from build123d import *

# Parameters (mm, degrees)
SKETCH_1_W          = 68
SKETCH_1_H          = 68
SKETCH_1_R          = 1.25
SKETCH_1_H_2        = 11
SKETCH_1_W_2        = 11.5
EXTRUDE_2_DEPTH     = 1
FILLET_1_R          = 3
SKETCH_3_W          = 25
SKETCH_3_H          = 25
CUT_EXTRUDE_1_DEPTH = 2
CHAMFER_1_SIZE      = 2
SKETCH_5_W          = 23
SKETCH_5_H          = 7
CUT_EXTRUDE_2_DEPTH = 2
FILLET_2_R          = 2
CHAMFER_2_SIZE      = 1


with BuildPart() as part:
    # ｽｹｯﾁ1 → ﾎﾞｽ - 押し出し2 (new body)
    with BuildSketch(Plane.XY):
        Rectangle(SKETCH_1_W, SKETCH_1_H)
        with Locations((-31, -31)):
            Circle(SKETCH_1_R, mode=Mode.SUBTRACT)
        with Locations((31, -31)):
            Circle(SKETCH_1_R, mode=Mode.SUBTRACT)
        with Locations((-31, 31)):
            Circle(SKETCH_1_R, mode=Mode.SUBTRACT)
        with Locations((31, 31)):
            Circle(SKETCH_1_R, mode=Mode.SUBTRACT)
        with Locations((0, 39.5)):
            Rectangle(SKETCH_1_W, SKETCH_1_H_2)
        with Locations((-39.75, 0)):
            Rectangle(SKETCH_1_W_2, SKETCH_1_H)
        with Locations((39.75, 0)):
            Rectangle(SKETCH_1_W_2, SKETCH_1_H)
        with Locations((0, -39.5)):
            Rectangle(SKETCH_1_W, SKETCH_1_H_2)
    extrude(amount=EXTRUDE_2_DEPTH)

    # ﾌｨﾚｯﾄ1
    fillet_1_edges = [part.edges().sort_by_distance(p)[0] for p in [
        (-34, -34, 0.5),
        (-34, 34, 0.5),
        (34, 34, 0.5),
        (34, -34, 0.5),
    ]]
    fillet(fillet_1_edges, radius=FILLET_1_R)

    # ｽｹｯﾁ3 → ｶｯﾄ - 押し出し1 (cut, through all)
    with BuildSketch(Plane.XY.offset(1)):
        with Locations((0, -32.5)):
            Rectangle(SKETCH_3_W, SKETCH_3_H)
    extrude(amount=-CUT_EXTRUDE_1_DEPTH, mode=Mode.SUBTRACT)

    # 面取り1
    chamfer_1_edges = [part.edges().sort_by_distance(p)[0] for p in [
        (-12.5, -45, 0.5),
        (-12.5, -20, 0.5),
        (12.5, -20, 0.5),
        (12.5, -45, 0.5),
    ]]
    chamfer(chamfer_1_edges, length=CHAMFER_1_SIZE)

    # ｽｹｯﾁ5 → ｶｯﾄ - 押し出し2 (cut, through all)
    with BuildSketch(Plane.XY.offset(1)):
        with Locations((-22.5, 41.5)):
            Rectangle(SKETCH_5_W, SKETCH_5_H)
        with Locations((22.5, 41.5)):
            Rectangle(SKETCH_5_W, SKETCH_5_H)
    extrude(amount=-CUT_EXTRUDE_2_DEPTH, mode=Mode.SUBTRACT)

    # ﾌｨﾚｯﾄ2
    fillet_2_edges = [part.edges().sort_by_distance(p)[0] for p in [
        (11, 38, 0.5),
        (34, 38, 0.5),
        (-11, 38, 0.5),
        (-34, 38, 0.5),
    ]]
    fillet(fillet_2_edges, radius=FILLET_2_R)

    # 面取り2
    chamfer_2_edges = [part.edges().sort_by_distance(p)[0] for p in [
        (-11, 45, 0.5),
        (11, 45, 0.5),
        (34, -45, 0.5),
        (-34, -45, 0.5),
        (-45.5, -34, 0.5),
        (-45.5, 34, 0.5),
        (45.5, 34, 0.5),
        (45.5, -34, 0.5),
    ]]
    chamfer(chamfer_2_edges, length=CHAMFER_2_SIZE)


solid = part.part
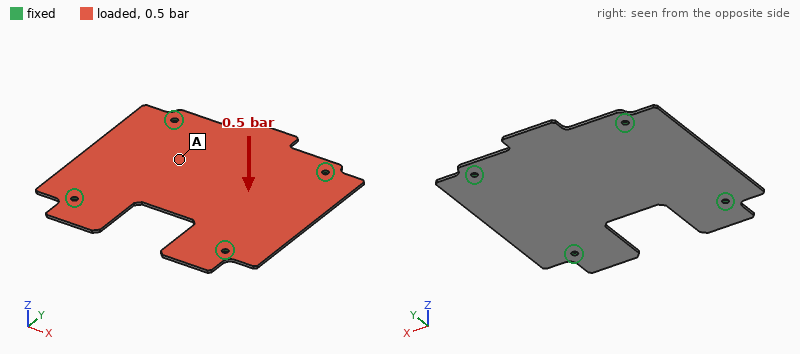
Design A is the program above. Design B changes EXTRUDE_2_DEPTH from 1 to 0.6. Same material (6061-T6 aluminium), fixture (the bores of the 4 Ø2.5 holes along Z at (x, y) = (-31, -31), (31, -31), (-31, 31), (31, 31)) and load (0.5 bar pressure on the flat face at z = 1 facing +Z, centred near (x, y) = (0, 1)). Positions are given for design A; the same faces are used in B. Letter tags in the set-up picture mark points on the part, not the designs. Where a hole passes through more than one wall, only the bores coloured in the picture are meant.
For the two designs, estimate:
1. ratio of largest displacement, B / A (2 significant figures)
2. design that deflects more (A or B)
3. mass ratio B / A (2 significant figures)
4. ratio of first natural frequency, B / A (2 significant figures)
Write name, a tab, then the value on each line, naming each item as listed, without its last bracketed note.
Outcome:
ratio of largest displacement, B / A	4.6
design that deflects more	B
mass ratio B / A	0.60
ratio of first natural frequency, B / A	0.61
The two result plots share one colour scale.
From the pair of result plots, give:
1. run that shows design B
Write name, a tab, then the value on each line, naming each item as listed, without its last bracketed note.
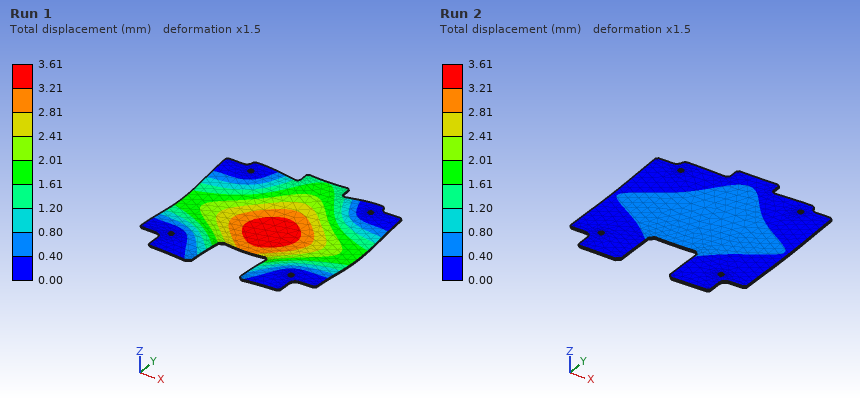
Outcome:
run that shows design B	Run 1
